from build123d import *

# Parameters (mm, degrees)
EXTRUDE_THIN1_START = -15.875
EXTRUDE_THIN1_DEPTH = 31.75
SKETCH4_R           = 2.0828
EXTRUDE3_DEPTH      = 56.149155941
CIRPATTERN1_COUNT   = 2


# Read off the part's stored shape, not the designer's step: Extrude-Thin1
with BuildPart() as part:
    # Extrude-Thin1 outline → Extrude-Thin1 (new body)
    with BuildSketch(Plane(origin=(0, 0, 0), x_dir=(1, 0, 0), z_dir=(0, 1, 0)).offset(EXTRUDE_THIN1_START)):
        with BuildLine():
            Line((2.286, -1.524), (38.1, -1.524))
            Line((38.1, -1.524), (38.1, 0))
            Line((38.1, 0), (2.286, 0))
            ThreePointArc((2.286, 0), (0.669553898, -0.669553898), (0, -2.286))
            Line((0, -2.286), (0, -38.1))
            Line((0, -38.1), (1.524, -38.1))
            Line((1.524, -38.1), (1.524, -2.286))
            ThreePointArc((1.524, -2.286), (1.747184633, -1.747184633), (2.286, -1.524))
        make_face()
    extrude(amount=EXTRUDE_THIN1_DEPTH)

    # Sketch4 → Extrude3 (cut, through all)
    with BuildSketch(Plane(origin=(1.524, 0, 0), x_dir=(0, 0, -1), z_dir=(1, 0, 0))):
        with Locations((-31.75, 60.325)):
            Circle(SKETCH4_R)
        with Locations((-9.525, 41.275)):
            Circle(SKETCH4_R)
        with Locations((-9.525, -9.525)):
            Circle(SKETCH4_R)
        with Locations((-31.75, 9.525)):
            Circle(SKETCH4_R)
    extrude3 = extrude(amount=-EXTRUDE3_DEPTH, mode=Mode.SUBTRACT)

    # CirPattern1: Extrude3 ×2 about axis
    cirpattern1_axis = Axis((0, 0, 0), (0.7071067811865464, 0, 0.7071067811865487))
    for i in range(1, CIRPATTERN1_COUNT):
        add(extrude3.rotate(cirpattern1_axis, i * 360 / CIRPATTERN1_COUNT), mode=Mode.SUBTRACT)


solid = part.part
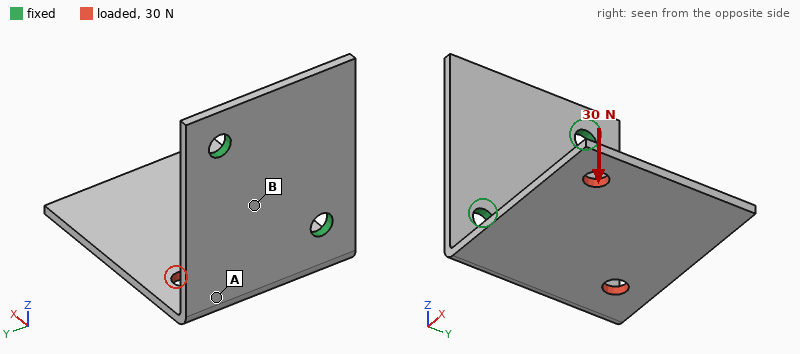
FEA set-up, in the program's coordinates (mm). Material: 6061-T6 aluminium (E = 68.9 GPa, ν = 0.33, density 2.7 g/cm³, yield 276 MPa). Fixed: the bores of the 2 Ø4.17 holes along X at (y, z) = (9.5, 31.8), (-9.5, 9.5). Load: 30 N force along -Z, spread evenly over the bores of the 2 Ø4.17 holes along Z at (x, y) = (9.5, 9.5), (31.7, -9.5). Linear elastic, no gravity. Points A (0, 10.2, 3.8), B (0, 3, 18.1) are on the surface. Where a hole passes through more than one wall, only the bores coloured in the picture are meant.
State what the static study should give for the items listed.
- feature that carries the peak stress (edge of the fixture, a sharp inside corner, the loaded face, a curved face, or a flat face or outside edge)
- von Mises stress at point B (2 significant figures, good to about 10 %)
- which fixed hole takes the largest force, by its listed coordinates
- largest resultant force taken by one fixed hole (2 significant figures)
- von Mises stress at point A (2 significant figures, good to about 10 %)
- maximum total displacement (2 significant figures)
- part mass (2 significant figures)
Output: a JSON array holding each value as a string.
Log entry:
["a flat face or outside edge", "8.5 MPa", "(-9.5, 9.5)", "20 N", "33 MPa", "0.67 mm", "9.4 g"]
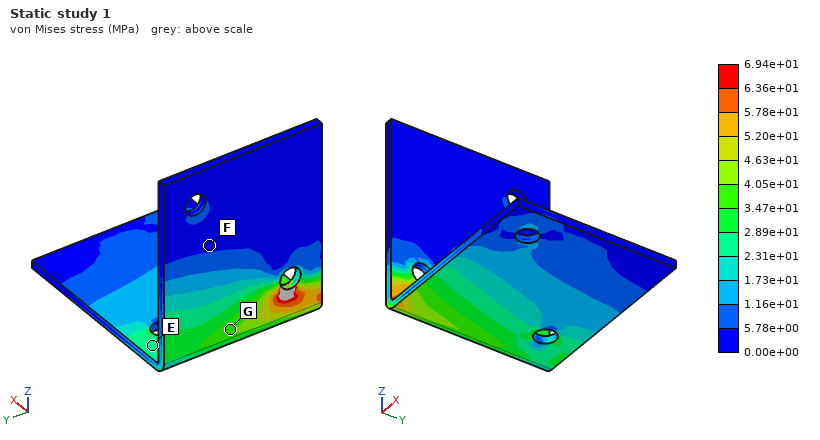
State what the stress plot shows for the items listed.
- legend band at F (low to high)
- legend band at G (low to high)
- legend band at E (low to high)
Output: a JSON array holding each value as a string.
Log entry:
["0.00e+00 to 5.78e+00 MPa", "3.47e+01 to 4.05e+01 MPa", "2.31e+01 to 2.89e+01 MPa"]
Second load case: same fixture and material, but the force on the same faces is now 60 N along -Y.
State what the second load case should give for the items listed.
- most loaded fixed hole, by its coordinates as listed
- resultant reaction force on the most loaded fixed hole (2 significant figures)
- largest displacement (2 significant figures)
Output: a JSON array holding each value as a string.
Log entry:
["(-9.5, 9.5)", "64 N", "0.46 mm"]
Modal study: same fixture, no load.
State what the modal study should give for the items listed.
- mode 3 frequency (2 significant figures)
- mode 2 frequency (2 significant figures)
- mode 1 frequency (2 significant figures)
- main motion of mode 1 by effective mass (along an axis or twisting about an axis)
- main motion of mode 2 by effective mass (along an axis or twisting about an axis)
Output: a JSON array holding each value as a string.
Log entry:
["2300 Hz", "1100 Hz", "630 Hz", "along Z", "along Y"]
